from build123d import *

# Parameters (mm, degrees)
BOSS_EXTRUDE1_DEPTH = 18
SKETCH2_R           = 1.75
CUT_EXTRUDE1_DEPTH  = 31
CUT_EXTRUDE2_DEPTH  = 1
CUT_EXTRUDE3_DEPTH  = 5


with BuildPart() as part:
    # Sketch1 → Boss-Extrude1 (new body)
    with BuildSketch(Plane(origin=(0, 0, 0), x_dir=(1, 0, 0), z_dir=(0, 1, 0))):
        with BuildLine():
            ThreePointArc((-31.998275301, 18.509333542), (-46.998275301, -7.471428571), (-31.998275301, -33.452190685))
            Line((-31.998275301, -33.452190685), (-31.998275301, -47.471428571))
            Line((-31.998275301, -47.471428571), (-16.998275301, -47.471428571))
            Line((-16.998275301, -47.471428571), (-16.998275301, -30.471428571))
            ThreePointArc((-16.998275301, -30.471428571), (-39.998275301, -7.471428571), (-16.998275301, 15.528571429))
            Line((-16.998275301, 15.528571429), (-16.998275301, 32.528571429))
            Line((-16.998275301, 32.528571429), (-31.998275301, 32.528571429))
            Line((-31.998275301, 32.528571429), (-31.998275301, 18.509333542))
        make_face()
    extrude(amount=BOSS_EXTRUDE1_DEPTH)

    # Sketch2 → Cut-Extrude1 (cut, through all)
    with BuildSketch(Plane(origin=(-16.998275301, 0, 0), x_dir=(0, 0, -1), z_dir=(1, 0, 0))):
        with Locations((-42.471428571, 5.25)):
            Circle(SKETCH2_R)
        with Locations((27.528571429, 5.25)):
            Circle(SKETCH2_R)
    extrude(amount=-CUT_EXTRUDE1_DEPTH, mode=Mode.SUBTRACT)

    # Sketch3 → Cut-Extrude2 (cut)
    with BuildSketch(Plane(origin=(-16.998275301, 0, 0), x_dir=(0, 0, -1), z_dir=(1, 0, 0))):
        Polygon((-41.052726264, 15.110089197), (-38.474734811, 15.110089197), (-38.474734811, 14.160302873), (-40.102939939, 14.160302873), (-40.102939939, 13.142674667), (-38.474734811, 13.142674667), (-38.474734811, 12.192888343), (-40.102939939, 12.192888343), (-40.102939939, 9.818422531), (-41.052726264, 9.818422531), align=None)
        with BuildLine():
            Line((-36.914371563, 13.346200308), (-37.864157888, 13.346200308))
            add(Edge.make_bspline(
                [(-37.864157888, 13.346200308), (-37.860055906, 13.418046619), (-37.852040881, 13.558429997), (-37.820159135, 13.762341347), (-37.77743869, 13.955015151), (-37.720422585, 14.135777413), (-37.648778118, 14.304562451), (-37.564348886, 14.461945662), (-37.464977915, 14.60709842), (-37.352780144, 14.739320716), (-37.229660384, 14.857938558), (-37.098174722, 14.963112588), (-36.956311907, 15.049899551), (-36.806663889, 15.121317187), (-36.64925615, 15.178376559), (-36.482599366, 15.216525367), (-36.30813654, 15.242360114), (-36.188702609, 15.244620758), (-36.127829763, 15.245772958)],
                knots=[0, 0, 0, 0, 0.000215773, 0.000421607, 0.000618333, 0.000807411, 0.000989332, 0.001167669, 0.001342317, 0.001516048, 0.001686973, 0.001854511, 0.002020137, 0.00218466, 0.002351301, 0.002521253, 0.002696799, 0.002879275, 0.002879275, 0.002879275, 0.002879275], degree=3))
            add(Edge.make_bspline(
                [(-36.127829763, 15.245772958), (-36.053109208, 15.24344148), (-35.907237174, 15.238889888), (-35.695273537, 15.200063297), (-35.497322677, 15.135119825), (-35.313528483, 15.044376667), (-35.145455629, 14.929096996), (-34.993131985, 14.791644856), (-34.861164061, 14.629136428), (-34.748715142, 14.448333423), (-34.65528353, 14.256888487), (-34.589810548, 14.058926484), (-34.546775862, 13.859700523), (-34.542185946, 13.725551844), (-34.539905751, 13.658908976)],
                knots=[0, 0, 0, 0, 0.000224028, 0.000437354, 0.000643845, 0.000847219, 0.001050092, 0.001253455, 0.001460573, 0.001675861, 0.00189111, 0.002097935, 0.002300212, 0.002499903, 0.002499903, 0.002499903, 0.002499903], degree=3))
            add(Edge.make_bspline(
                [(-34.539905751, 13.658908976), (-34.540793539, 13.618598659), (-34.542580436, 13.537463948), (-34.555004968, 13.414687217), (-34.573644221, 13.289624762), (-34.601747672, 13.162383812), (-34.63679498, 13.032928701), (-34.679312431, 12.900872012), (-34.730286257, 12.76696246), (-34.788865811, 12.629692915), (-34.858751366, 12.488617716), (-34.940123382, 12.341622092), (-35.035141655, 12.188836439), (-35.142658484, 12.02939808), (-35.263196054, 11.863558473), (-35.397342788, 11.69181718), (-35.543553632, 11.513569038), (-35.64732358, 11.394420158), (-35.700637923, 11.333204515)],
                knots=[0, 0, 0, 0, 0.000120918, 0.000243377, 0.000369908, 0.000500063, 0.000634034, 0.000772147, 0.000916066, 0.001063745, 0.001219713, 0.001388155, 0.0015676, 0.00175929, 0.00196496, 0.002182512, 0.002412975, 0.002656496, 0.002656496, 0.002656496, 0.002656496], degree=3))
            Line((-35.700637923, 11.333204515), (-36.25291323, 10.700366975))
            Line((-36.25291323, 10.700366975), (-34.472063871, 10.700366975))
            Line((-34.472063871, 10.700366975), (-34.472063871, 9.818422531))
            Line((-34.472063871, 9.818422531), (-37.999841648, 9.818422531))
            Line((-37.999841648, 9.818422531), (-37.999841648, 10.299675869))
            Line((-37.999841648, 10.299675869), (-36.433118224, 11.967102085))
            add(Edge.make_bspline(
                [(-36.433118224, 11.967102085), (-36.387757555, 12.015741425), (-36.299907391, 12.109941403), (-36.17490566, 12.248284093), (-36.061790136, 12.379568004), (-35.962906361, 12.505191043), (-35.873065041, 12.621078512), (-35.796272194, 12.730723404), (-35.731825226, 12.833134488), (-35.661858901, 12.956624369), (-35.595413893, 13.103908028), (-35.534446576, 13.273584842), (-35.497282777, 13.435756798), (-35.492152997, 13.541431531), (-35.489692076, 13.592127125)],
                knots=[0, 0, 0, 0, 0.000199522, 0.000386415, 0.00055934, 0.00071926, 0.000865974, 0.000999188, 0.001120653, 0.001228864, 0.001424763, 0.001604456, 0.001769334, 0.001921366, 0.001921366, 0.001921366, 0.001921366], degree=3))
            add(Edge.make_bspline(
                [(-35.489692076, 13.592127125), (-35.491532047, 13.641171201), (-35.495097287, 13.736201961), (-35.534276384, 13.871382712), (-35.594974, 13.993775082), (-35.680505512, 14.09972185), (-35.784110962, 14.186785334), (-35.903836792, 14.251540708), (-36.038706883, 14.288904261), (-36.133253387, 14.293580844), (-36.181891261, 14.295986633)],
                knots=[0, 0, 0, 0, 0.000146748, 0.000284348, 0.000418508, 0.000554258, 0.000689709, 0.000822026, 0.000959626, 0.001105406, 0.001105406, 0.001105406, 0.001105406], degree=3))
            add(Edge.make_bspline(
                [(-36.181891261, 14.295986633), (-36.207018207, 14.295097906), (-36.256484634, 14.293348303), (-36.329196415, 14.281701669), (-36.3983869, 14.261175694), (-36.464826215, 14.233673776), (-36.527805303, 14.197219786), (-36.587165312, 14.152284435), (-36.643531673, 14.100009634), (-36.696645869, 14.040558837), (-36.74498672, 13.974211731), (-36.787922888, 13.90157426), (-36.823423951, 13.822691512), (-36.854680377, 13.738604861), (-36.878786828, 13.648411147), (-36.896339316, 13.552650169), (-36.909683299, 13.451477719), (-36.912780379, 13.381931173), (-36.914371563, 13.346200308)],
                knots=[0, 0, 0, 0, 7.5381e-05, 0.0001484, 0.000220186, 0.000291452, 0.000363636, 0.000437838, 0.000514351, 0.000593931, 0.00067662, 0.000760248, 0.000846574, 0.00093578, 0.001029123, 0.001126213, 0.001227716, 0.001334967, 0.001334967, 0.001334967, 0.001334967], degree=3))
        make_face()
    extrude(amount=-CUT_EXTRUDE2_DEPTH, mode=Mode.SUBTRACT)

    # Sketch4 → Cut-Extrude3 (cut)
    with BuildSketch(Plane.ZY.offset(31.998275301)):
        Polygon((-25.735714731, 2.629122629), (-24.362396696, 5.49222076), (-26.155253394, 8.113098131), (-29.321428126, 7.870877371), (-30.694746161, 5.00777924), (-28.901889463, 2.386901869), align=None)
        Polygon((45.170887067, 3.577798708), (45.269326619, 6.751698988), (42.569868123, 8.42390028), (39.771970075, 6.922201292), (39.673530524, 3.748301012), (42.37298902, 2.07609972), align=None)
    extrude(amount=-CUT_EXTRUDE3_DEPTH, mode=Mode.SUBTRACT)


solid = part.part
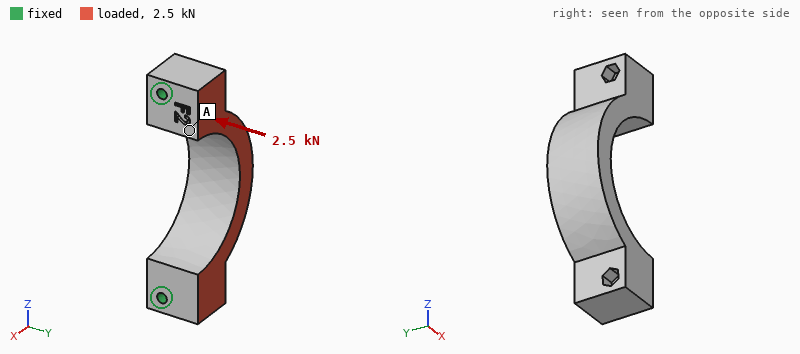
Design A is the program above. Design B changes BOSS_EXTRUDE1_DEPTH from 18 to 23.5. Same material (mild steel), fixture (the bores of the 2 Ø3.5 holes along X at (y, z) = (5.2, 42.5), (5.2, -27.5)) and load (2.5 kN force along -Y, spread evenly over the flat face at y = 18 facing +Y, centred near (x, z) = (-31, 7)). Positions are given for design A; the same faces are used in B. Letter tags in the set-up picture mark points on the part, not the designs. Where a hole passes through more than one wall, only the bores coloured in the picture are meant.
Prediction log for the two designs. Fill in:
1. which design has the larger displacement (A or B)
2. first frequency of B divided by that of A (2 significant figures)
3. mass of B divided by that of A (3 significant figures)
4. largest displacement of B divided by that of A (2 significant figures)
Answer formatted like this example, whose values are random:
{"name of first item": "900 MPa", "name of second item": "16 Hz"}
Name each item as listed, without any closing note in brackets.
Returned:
{"which design has the larger displacement": "A", "first frequency of B divided by that of A": "0.89", "mass of B divided by that of A": "1.31", "largest displacement of B divided by that of A": "0.92"}
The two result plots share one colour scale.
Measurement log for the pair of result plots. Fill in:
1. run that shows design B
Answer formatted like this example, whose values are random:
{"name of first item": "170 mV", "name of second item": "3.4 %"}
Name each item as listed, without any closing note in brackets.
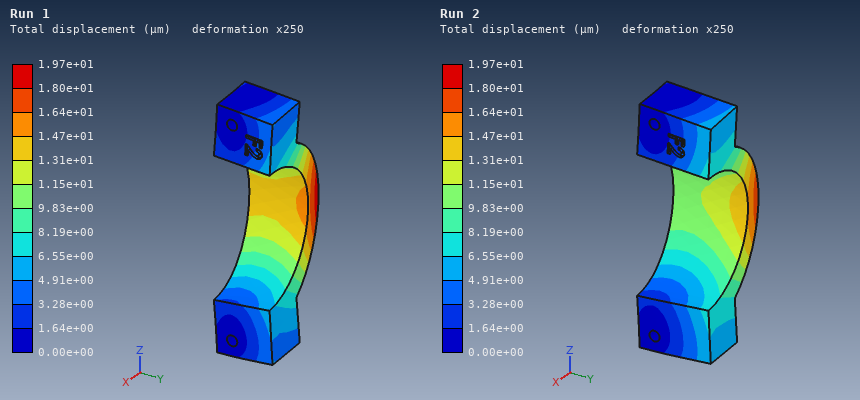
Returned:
{"run that shows design B": "Run 2"}
